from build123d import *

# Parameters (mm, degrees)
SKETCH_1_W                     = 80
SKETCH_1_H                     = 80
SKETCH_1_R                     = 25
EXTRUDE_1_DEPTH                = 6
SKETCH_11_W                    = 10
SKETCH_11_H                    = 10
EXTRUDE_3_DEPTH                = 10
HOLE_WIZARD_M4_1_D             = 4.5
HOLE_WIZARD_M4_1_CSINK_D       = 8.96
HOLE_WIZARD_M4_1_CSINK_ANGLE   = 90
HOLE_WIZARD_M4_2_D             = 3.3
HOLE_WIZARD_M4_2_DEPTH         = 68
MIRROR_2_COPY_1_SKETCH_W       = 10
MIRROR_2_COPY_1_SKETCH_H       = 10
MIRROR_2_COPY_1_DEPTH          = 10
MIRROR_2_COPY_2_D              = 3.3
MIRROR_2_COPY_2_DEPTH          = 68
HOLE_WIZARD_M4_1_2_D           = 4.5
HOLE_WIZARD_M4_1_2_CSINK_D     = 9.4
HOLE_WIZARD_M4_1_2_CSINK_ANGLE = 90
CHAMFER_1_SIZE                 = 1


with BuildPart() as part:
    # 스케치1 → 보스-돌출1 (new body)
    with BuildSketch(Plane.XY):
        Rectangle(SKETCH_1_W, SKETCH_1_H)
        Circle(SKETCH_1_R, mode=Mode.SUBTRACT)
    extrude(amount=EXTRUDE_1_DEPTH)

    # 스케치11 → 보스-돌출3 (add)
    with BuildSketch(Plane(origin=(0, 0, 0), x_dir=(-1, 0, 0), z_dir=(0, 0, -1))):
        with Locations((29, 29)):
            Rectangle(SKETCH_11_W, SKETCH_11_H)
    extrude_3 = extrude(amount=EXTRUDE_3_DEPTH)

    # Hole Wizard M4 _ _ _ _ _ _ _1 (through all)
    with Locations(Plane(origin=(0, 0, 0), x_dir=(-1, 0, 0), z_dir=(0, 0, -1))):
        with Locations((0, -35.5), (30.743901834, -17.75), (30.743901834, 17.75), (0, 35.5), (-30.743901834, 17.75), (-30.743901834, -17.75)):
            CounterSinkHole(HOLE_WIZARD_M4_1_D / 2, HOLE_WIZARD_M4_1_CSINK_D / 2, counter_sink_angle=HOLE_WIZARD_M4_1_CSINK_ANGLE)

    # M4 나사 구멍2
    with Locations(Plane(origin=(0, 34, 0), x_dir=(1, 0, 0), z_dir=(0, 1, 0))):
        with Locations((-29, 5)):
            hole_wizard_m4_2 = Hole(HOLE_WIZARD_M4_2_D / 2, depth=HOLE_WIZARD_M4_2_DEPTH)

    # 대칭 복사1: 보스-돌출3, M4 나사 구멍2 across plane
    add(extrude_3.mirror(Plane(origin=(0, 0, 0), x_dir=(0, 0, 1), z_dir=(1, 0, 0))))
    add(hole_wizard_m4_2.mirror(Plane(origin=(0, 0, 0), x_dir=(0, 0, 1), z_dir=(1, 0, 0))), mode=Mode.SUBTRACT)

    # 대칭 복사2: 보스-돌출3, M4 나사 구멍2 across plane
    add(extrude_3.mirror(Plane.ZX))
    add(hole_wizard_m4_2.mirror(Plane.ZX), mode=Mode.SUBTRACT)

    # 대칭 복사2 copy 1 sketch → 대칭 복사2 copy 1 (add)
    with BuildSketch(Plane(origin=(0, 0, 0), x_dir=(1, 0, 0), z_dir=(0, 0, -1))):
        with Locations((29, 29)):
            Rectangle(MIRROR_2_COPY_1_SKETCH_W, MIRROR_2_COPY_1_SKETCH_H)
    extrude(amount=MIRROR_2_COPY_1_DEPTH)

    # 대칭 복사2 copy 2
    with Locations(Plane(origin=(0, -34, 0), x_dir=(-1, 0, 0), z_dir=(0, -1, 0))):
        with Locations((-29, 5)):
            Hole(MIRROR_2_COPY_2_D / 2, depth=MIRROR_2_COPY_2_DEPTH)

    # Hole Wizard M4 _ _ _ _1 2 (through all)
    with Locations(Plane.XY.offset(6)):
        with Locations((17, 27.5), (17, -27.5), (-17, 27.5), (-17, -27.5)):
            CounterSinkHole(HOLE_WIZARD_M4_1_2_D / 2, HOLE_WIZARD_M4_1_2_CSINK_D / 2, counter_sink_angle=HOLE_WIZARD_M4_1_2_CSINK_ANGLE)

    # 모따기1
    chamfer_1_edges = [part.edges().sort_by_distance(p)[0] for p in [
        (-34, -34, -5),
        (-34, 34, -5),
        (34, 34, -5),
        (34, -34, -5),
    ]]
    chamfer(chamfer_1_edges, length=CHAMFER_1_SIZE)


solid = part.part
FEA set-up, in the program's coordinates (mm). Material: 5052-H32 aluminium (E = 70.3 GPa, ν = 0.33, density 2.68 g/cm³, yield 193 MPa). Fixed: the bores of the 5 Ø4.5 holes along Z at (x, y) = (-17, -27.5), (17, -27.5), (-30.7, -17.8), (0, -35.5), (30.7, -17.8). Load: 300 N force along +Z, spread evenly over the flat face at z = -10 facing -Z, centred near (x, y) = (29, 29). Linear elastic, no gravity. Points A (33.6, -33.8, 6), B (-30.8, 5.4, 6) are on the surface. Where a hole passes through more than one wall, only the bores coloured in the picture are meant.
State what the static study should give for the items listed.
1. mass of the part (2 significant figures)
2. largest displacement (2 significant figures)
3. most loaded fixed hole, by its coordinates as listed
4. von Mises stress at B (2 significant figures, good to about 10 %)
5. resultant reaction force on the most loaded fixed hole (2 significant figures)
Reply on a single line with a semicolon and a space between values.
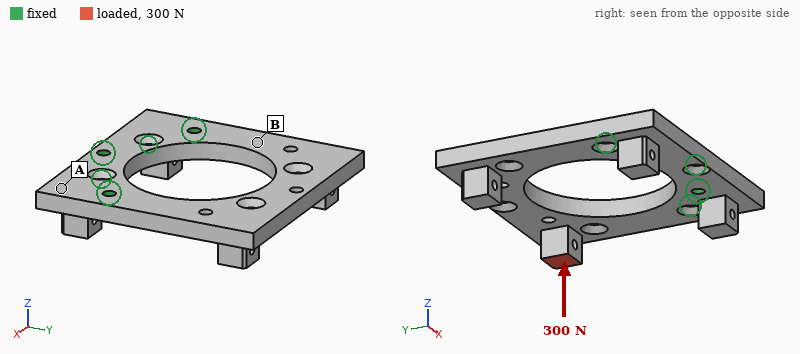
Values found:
77 g; 0.50 mm; (30.7, -17.8); 35 MPa; 500 N
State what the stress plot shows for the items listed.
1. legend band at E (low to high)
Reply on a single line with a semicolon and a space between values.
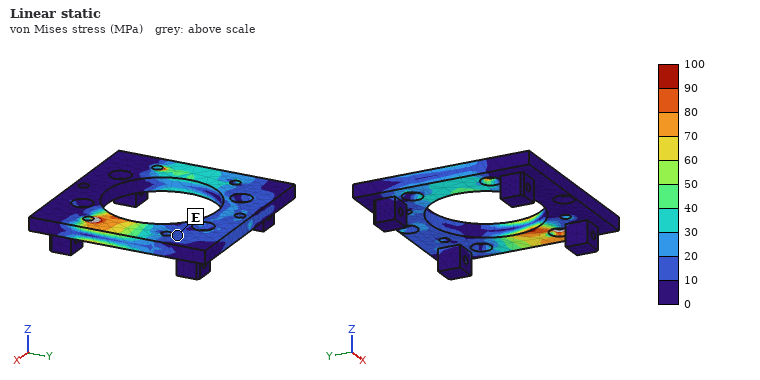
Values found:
10 to 20 MPa
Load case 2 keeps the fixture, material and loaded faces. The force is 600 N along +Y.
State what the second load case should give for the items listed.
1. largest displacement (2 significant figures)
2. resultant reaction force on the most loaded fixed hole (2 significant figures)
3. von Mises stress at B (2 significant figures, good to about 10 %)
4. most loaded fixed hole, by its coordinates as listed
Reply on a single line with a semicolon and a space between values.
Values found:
0.42 mm; 450 N; 31 MPa; (30.7, -17.8)
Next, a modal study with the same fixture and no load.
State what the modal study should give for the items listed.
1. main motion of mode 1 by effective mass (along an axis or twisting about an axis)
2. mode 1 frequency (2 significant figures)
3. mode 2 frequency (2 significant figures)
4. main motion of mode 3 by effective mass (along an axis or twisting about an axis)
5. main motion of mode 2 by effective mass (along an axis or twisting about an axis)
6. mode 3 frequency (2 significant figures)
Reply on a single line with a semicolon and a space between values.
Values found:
along Z; 890 Hz; 1900 Hz; along X; twisting about Y; 4500 Hz
